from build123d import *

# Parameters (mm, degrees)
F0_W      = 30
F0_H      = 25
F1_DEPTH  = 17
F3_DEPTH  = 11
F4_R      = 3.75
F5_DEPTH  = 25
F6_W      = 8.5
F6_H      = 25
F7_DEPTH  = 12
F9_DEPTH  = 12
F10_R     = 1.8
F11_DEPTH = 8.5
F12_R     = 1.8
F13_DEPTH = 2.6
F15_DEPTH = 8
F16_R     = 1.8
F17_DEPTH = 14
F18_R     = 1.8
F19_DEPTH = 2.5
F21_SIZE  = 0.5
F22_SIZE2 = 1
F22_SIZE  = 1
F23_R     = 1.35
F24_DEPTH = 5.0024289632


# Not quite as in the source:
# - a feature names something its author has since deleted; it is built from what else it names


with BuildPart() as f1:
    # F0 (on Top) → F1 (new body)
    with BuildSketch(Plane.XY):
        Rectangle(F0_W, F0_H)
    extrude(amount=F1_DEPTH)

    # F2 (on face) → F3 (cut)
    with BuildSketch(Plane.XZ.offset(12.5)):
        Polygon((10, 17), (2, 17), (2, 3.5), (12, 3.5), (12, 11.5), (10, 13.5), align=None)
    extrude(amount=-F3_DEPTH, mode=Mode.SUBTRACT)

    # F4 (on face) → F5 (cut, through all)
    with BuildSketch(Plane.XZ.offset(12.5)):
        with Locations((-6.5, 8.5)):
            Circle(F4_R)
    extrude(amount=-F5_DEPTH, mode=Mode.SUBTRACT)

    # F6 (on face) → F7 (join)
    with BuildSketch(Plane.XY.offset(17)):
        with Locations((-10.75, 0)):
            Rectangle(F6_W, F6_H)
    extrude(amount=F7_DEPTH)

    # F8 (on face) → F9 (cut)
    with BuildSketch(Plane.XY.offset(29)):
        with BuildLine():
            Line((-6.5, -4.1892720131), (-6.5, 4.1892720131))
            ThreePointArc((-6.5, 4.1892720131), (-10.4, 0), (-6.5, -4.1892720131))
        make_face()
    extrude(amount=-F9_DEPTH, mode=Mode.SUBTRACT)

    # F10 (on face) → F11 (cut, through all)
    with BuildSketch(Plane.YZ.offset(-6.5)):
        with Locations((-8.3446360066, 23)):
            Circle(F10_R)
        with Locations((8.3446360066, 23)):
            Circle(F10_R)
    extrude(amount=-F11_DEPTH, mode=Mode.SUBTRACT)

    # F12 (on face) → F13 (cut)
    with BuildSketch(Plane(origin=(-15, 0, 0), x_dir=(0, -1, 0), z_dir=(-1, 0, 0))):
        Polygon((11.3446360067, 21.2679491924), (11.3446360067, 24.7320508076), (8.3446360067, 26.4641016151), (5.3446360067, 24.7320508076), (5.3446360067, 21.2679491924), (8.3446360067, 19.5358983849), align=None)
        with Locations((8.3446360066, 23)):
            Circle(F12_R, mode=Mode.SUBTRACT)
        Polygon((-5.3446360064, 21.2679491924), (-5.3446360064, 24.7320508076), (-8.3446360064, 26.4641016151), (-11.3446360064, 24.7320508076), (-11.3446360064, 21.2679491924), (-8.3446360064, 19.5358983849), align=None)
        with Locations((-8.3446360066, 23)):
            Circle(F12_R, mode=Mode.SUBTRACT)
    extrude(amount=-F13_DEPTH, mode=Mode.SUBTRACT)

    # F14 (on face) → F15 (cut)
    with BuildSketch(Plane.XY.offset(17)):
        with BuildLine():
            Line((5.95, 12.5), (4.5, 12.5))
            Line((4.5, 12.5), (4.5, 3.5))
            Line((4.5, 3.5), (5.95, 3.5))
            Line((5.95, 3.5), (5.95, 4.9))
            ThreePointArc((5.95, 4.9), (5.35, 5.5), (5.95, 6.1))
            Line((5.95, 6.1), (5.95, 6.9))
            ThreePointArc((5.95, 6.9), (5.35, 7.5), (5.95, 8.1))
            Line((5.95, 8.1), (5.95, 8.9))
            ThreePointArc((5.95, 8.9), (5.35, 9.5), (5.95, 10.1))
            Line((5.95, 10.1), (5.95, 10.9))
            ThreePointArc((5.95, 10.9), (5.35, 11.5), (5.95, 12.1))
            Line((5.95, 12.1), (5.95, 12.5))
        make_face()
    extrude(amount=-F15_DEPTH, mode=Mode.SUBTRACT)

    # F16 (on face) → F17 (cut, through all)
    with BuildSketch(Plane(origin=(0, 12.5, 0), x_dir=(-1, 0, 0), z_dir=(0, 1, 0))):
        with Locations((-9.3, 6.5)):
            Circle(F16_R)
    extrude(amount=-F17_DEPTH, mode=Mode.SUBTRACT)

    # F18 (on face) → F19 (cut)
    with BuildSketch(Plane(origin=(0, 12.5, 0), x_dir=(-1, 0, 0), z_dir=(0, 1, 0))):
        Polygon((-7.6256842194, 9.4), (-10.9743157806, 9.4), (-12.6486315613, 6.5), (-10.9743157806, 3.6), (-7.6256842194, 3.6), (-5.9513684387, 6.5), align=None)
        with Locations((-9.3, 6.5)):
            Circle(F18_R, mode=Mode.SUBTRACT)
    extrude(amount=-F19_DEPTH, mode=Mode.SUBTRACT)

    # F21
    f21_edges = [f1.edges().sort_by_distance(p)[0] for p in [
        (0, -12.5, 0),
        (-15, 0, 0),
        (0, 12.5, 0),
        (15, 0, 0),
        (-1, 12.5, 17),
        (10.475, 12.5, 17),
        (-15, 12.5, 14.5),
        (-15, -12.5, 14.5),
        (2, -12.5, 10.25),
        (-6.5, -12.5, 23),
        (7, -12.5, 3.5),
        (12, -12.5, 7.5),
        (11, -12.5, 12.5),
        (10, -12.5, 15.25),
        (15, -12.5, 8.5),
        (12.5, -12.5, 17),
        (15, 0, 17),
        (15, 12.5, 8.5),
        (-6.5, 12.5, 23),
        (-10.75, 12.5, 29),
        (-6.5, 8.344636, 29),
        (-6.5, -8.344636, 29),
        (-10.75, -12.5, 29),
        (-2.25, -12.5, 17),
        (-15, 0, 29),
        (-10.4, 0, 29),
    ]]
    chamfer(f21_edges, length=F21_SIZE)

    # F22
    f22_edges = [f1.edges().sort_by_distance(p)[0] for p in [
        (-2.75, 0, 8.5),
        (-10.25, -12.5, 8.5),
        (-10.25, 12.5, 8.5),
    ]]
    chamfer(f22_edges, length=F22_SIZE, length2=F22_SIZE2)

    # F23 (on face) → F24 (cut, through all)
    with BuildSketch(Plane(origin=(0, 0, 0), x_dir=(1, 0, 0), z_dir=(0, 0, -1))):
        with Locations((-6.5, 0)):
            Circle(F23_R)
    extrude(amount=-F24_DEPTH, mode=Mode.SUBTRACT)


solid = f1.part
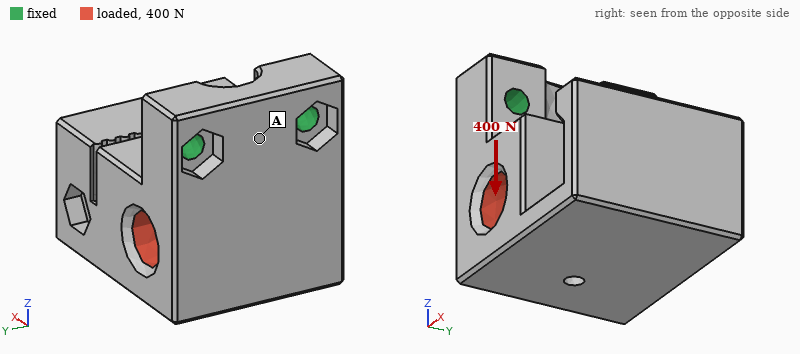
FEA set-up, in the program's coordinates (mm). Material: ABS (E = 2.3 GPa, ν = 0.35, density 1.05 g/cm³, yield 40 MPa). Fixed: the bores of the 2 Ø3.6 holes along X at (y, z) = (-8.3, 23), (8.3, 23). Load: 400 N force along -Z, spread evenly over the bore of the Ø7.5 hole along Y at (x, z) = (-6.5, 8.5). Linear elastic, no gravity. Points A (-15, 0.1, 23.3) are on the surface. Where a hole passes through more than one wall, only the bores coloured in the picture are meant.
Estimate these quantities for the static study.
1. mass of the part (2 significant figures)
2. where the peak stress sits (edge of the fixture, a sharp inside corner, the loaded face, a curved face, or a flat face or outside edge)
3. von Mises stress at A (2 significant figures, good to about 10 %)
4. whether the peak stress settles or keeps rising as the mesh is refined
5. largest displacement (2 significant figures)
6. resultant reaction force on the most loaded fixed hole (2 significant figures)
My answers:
12 g
edge of the fixture
2.1 MPa
keeps rising
0.29 mm
200 N
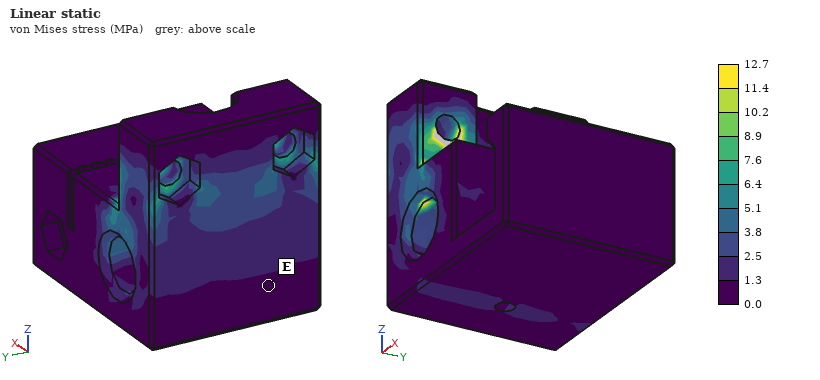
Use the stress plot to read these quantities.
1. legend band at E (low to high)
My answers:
0.0 to 1.3 MPa
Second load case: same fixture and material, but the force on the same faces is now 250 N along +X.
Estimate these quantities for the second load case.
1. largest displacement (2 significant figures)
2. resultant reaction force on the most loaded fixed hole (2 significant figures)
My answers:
0.53 mm
130 N
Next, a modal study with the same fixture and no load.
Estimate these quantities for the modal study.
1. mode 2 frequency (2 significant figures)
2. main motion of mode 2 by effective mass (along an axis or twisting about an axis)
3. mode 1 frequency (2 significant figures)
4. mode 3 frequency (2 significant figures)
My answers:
2100 Hz
along Y
1100 Hz
4300 Hz
